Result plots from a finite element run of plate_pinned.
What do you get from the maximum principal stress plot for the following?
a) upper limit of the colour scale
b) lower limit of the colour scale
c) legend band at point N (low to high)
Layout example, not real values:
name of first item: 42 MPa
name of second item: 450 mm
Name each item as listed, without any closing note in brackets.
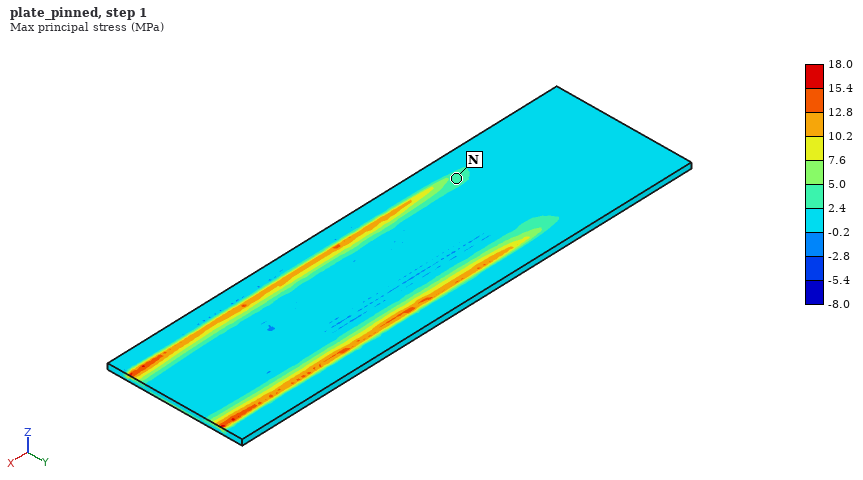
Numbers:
upper limit of the colour scale: 18.0 MPa
lower limit of the colour scale: -8.0 MPa
legend band at point N: 2.4 to 5.0 MPa
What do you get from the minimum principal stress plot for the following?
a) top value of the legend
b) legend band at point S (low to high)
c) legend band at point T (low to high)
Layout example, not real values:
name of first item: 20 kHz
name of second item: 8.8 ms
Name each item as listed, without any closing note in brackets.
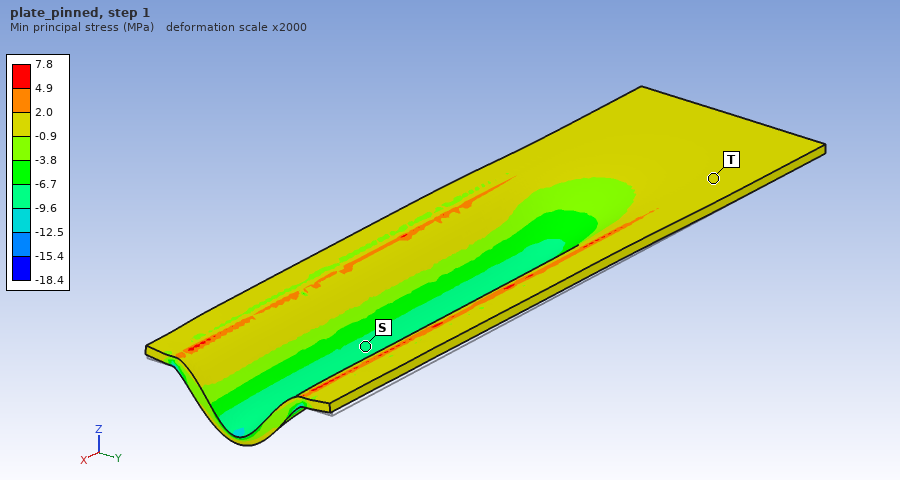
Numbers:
top value of the legend: 7.8 MPa
legend band at point S: -9.6 to -6.7 MPa
legend band at point T: -0.9 to 2.0 MPa
